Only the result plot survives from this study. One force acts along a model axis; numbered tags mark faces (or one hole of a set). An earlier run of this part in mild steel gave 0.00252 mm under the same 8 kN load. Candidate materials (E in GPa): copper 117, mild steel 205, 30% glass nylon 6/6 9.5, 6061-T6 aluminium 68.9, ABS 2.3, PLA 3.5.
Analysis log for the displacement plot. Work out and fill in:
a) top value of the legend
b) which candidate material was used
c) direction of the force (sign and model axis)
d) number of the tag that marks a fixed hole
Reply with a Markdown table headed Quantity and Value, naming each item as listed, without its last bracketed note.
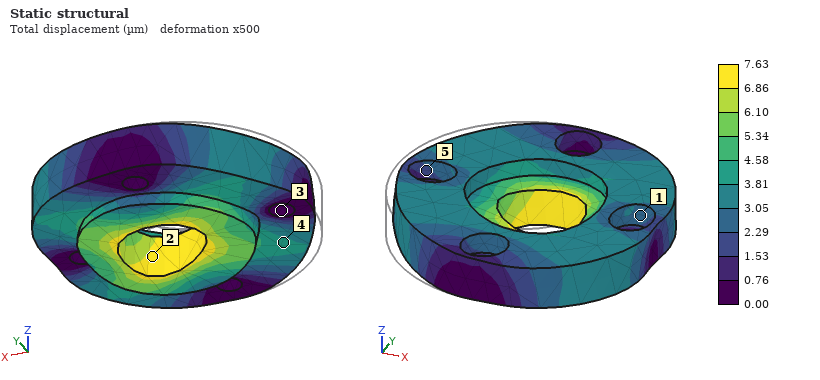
| Quantity | Value |
|---|---|
| top value of the legend | 7.63 µm |
| which candidate material was used | 6061-T6 aluminium |
| direction of the force | +X |
| number of the tag that marks a fixed hole | 3 |
